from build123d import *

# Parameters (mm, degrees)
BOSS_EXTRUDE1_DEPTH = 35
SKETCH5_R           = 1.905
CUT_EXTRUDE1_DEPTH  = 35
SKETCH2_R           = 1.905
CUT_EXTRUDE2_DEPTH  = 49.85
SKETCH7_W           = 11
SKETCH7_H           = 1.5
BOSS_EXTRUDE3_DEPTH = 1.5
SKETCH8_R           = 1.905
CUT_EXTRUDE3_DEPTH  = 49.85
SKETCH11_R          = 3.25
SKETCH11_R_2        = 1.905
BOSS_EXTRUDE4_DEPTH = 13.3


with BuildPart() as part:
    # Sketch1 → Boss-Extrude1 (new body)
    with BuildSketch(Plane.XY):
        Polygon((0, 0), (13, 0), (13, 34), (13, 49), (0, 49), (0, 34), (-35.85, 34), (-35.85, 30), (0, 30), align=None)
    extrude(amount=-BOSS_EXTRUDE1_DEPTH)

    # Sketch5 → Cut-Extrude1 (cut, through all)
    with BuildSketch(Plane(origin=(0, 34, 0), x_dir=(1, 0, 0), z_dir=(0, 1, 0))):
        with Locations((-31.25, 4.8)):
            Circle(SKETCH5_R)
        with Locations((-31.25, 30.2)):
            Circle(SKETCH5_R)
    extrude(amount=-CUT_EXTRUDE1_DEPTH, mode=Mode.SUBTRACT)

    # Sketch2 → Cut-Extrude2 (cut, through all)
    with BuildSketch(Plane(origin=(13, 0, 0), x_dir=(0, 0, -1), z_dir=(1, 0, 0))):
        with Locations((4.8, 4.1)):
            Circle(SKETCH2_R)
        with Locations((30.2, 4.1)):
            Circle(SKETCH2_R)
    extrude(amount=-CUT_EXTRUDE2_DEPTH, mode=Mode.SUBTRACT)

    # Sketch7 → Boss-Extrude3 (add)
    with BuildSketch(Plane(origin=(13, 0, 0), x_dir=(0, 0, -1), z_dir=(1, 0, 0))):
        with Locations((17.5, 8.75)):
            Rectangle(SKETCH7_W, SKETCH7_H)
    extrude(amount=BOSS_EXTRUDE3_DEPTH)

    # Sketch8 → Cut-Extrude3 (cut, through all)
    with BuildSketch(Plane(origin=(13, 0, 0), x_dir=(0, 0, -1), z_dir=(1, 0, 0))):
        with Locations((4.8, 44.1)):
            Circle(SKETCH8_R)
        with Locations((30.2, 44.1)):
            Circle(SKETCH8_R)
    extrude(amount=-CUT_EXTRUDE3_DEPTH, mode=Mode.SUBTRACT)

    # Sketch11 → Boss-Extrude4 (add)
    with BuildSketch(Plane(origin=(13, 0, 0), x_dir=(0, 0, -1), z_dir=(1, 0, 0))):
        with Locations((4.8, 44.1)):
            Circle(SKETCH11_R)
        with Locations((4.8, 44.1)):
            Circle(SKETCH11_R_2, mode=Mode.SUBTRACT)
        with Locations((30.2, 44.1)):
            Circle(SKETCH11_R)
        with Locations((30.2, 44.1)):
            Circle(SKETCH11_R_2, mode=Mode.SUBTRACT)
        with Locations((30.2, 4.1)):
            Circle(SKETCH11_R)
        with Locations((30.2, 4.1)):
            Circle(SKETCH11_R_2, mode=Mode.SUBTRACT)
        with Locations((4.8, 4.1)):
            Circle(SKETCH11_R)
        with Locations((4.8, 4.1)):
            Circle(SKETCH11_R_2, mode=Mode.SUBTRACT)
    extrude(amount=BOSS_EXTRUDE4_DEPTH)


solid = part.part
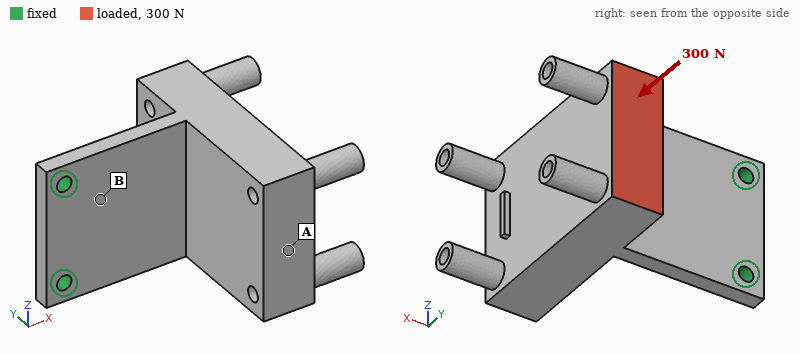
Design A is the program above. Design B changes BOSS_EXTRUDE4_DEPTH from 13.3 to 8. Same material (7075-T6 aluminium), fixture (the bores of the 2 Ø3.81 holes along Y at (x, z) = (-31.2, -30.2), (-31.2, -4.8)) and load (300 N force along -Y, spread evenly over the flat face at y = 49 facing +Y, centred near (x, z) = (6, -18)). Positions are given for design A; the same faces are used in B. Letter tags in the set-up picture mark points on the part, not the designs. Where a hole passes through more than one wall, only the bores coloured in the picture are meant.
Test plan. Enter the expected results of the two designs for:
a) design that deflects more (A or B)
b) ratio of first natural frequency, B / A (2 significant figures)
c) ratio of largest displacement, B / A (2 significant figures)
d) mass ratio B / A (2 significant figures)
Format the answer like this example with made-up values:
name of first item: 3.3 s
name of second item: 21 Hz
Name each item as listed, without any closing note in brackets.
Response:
design that deflects more: A
ratio of first natural frequency, B / A: 1.0
ratio of largest displacement, B / A: 0.92
mass ratio B / A: 0.98
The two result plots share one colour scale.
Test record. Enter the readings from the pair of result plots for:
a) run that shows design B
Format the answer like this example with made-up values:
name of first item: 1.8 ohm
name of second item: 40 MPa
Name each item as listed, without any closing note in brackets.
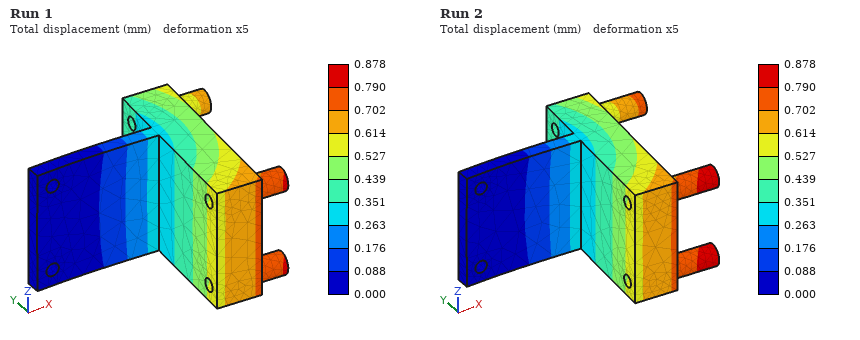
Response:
run that shows design B: Run 1
